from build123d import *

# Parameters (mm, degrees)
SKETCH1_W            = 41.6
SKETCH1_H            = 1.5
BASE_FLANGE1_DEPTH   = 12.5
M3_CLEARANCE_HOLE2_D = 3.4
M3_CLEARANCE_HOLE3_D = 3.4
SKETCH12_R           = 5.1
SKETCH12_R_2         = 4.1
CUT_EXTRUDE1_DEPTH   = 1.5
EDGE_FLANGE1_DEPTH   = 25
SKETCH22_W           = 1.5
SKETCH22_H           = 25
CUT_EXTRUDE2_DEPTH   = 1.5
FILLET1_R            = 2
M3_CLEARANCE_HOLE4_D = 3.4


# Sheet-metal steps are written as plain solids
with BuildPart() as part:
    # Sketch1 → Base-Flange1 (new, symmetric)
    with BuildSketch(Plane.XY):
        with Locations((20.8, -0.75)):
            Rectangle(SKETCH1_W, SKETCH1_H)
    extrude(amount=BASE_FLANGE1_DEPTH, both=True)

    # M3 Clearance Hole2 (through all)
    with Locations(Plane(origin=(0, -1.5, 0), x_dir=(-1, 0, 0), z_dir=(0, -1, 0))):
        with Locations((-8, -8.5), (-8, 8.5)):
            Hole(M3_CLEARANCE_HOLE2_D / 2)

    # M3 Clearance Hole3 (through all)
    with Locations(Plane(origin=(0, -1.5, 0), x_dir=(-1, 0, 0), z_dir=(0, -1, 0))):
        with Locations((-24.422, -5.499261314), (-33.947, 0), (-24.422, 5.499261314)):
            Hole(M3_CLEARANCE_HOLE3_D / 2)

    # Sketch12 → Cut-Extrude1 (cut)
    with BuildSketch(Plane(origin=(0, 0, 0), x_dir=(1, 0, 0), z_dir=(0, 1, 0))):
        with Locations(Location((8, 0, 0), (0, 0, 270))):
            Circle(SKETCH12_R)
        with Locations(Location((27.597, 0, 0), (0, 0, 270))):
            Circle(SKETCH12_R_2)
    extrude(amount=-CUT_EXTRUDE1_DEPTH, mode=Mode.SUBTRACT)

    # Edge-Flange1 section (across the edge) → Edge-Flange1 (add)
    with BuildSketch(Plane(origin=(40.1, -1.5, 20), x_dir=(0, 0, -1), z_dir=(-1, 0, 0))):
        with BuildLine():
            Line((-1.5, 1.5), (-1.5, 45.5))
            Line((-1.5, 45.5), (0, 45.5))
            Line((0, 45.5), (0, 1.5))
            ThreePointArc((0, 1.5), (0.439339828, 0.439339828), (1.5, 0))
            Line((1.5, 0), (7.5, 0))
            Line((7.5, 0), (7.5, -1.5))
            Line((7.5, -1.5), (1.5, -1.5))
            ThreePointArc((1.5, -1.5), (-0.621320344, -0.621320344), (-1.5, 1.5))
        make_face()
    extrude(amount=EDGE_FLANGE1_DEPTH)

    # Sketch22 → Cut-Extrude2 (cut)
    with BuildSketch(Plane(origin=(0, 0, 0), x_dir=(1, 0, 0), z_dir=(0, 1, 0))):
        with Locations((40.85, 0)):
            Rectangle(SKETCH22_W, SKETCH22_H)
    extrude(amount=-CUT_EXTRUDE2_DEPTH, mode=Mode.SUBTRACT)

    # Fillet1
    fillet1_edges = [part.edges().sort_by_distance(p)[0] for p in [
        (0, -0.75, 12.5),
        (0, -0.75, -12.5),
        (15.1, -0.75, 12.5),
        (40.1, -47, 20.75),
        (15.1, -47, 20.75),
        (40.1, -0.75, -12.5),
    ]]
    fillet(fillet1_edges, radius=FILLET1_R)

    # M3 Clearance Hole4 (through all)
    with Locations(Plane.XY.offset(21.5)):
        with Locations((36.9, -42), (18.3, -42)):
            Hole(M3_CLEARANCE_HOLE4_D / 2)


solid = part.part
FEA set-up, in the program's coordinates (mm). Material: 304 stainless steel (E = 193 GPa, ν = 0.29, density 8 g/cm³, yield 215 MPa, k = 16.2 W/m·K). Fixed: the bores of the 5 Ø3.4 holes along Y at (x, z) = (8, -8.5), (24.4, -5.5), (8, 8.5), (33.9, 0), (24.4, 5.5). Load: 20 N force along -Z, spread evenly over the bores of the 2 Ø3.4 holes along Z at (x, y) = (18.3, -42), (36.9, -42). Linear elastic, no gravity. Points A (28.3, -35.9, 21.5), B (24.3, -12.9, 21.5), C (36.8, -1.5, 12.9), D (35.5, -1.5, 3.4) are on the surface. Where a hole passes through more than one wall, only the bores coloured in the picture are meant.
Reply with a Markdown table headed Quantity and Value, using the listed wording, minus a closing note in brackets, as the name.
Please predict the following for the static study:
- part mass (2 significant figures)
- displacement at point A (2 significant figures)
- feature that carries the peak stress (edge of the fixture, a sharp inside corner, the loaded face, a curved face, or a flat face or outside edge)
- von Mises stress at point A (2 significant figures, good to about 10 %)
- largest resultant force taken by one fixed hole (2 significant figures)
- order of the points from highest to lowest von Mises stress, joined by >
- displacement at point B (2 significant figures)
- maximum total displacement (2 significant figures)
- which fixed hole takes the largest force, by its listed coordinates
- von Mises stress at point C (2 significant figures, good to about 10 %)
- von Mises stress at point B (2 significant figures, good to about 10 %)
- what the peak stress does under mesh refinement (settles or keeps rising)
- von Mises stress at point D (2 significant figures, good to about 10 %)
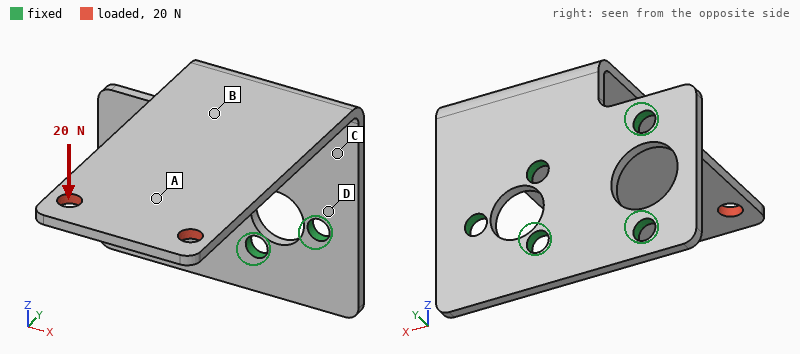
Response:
| Quantity | Value |
|---|---|
| part mass | 26 g |
| displacement at point A | 0.54 mm |
| feature that carries the peak stress | edge of the fixture |
| von Mises stress at point A | 13 MPa |
| largest resultant force taken by one fixed hole | 30 N |
| order of the points from highest to lowest von Mises stress, joined by > | C > B > D > A |
| displacement at point B | 0.15 mm |
| maximum total displacement | 0.76 mm |
| which fixed hole takes the largest force, by its listed coordinates | (24.4, 5.5) |
| von Mises stress at point C | 73 MPa |
| von Mises stress at point B | 57 MPa |
| what the peak stress does under mesh refinement | keeps rising |
| von Mises stress at point D | 39 MPa |
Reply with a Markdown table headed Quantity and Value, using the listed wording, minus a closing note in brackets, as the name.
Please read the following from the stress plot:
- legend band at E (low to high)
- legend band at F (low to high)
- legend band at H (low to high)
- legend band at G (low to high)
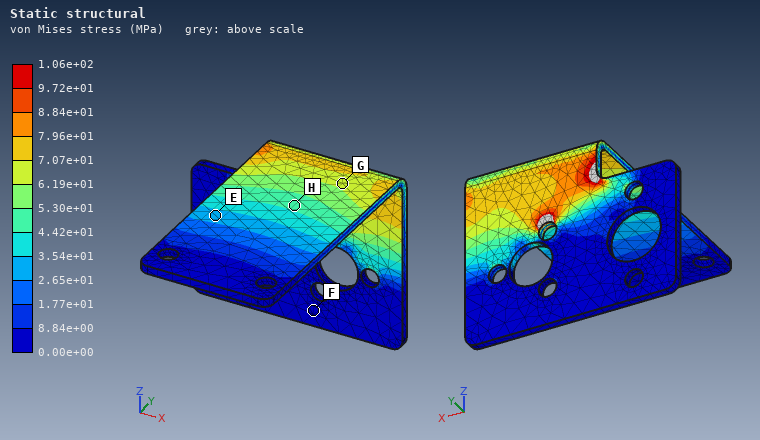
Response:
| Quantity | Value |
|---|---|
| legend band at E | 2.65e+01 to 3.54e+01 MPa |
| legend band at F | 0.00e+00 to 8.84e+00 MPa |
| legend band at H | 4.42e+01 to 5.30e+01 MPa |
| legend band at G | 6.19e+01 to 7.07e+01 MPa |
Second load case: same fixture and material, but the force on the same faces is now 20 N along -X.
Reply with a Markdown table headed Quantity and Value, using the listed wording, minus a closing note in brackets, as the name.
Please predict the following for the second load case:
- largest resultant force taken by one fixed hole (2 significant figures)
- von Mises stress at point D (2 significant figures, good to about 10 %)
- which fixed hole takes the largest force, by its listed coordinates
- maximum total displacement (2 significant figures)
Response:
| Quantity | Value |
|---|---|
| largest resultant force taken by one fixed hole | 34 N |
| von Mises stress at point D | 53 MPa |
| which fixed hole takes the largest force, by its listed coordinates | (8, 8.5) |
| maximum total displacement | 0.17 mm |
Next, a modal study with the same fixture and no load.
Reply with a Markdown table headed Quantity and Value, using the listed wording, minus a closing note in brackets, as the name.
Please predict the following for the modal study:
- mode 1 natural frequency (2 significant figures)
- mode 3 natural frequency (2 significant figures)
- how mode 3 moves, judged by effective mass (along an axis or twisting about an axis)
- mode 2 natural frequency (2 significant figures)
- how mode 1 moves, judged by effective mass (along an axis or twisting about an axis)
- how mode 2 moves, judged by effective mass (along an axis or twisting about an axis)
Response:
| Quantity | Value |
|---|---|
| mode 1 natural frequency | 390 Hz |
| mode 3 natural frequency | 1900 Hz |
| how mode 3 moves, judged by effective mass | along Y |
| mode 2 natural frequency | 780 Hz |
| how mode 1 moves, judged by effective mass | along Z |
| how mode 2 moves, judged by effective mass | along X |
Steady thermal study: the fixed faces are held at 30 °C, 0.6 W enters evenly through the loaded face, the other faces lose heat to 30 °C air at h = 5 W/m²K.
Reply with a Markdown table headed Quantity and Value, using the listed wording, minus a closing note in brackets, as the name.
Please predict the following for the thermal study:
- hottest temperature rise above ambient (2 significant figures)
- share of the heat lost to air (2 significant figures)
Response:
| Quantity | Value |
|---|---|
| hottest temperature rise above ambient | 40 K |
| share of the heat lost to air | 48 % |
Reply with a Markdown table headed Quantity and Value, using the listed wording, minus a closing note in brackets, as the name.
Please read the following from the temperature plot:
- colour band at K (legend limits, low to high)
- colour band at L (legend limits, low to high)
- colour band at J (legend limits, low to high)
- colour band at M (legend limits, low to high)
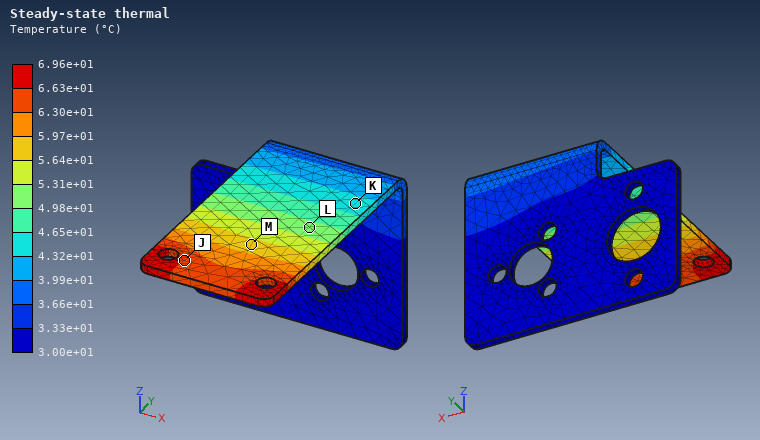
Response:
| Quantity | Value |
|---|---|
| colour band at K | 4.32e+01 to 4.65e+01 °C |
| colour band at L | 4.98e+01 to 5.31e+01 °C |
| colour band at J | 6.30e+01 to 6.63e+01 °C |
| colour band at M | 5.64e+01 to 5.97e+01 °C |
